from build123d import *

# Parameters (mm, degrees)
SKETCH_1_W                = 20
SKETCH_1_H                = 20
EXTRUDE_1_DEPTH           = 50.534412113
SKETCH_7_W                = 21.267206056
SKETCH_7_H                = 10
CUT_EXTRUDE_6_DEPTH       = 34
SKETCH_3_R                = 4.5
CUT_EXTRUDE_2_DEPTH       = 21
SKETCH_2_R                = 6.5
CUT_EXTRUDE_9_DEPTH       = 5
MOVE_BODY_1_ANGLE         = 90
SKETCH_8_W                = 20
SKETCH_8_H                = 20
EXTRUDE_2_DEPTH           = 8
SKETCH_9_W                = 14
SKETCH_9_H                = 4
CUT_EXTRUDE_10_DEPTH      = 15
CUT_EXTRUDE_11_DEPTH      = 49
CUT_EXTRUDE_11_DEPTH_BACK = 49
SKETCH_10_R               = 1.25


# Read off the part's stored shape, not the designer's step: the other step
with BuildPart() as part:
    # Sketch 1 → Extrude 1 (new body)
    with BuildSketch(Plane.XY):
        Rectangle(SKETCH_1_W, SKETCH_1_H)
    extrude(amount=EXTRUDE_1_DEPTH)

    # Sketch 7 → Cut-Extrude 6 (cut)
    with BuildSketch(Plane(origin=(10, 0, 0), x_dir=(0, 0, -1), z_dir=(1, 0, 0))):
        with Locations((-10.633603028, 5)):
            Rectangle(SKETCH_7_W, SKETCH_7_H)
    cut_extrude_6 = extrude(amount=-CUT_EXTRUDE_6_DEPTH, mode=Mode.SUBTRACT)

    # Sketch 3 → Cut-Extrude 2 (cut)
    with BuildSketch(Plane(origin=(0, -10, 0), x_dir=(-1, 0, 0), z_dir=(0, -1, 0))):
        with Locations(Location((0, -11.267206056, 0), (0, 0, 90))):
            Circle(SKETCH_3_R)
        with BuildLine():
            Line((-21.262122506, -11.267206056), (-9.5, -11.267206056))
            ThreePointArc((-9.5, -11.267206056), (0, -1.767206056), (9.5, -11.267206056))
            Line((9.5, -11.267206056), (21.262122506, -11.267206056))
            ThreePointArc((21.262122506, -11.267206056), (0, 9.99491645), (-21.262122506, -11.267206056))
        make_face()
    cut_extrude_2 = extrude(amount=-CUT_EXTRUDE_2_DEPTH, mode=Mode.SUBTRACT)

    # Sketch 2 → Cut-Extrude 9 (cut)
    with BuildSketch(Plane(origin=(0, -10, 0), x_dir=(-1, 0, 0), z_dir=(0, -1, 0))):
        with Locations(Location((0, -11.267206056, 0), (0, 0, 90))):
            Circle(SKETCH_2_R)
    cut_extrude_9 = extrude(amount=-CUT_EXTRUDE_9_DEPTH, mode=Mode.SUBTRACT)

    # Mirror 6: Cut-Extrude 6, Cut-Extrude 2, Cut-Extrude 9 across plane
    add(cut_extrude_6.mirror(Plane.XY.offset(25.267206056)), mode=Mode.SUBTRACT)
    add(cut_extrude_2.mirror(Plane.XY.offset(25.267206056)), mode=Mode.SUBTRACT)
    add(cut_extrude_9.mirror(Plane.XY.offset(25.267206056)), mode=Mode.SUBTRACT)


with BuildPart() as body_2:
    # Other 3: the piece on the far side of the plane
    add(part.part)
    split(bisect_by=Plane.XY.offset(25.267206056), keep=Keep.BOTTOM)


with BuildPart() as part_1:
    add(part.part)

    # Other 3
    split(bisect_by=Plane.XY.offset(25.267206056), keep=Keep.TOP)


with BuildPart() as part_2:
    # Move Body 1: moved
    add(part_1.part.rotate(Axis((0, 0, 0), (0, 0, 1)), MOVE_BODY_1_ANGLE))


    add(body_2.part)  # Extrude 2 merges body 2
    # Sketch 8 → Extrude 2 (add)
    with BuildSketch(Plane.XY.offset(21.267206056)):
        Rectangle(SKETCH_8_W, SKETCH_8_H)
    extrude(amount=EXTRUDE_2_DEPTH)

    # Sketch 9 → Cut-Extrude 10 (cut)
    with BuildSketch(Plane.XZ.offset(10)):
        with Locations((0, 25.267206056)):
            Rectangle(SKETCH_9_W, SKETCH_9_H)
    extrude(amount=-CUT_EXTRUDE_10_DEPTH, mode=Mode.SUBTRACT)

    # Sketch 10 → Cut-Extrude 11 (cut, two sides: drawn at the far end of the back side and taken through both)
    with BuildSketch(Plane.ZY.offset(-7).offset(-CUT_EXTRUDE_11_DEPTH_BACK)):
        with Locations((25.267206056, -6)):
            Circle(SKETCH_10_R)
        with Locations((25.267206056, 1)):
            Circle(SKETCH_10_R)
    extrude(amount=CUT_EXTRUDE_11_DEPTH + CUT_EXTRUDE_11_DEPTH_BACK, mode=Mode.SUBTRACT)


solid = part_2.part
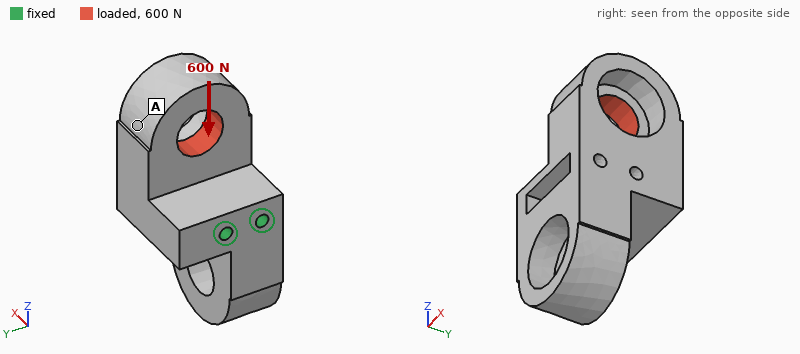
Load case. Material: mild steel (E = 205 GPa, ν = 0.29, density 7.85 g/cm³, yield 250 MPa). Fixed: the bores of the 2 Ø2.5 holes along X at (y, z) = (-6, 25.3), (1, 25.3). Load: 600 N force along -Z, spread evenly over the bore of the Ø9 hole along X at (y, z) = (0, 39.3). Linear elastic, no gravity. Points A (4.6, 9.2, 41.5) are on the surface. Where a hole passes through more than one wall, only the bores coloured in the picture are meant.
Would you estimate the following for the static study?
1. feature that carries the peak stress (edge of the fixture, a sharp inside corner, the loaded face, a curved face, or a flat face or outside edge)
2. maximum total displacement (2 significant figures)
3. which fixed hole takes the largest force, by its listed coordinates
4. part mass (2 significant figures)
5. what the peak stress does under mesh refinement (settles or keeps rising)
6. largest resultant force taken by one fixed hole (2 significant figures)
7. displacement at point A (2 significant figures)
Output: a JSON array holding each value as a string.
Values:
["edge of the fixture", "35 µm", "(1, 25.3)", "56 g", "keeps rising", "420 N", "25 µm"]
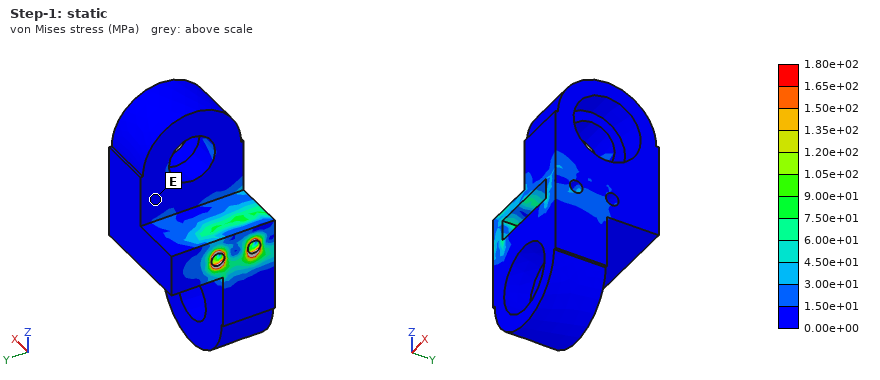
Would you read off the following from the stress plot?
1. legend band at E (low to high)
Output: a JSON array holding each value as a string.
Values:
["0.00e+00 to 1.50e+01 MPa"]
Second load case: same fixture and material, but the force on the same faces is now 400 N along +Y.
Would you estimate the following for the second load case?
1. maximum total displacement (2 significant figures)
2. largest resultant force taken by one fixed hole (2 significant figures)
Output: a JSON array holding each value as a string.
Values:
["20 µm", "750 N"]
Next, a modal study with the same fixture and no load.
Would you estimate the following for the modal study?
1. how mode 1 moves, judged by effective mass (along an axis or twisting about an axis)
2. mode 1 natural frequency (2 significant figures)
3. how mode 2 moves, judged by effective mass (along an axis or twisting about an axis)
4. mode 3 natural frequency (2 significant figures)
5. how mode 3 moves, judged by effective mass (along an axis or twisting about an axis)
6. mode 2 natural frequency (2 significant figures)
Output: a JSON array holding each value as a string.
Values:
["along Z", "3000 Hz", "along Y", "7600 Hz", "along Y", "5800 Hz"]
